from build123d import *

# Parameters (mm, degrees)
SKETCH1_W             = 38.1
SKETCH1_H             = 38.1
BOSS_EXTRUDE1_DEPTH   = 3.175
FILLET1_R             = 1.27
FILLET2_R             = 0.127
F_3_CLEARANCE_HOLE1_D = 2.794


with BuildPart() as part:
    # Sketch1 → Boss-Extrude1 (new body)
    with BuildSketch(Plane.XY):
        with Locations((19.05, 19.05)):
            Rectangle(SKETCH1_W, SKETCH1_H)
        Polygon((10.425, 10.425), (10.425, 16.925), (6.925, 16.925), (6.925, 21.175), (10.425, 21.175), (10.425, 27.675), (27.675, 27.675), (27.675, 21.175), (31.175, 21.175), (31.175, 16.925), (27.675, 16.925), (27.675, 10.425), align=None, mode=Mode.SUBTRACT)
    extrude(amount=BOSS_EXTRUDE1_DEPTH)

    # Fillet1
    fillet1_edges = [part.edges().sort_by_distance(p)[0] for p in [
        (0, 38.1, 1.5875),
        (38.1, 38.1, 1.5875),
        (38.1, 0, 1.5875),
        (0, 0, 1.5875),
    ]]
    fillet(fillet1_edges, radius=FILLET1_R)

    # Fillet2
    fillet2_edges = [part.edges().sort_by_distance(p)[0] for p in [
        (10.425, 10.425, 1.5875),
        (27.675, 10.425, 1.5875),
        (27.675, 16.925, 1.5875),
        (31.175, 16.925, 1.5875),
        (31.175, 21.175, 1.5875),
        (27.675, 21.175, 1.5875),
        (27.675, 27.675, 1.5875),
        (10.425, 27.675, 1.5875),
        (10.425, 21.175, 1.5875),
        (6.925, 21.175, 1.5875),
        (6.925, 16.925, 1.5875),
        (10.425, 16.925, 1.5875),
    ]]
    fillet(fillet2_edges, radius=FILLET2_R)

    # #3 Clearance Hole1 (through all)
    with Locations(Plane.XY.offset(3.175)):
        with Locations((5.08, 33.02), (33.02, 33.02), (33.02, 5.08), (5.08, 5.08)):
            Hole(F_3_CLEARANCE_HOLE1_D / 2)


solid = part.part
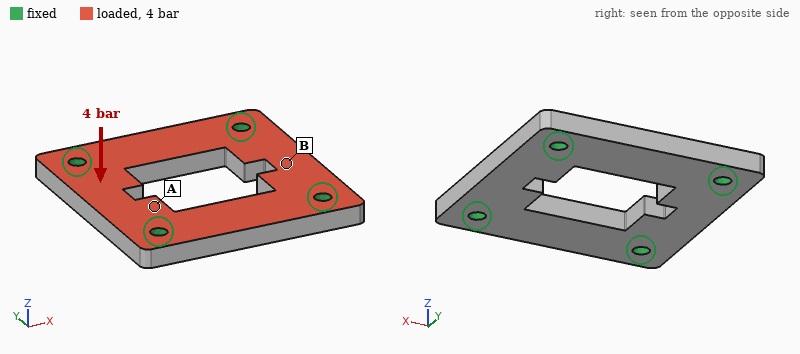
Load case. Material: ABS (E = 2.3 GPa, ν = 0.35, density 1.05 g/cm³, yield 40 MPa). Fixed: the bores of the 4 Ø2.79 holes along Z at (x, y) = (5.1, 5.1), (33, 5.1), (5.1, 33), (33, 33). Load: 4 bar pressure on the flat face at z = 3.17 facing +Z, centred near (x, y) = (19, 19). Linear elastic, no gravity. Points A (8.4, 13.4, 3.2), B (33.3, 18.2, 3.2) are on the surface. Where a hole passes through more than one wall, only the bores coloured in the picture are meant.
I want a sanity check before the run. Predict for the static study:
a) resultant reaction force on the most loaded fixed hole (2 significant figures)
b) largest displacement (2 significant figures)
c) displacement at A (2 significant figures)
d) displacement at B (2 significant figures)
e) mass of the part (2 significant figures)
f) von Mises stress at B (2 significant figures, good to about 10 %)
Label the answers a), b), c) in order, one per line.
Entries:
a) 110 N
b) 0.14 mm
c) 0.095 mm
d) 0.11 mm
e) 3.7 g
f) 7.4 MPa
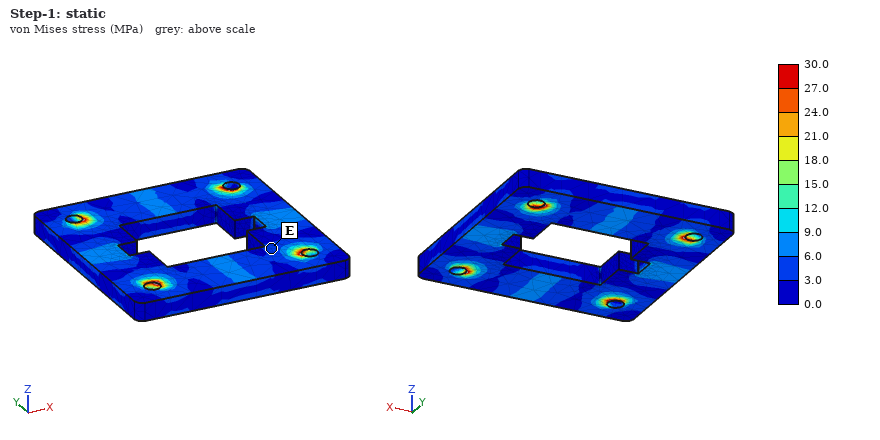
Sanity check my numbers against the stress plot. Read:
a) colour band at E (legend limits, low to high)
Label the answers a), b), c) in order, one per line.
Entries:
a) 3.0 to 6.0 MPa
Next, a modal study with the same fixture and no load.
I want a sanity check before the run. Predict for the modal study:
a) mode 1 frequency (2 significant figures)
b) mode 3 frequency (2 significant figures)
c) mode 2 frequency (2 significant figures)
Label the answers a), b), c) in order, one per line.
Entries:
a) 5800 Hz
b) 6100 Hz
c) 6100 Hz
